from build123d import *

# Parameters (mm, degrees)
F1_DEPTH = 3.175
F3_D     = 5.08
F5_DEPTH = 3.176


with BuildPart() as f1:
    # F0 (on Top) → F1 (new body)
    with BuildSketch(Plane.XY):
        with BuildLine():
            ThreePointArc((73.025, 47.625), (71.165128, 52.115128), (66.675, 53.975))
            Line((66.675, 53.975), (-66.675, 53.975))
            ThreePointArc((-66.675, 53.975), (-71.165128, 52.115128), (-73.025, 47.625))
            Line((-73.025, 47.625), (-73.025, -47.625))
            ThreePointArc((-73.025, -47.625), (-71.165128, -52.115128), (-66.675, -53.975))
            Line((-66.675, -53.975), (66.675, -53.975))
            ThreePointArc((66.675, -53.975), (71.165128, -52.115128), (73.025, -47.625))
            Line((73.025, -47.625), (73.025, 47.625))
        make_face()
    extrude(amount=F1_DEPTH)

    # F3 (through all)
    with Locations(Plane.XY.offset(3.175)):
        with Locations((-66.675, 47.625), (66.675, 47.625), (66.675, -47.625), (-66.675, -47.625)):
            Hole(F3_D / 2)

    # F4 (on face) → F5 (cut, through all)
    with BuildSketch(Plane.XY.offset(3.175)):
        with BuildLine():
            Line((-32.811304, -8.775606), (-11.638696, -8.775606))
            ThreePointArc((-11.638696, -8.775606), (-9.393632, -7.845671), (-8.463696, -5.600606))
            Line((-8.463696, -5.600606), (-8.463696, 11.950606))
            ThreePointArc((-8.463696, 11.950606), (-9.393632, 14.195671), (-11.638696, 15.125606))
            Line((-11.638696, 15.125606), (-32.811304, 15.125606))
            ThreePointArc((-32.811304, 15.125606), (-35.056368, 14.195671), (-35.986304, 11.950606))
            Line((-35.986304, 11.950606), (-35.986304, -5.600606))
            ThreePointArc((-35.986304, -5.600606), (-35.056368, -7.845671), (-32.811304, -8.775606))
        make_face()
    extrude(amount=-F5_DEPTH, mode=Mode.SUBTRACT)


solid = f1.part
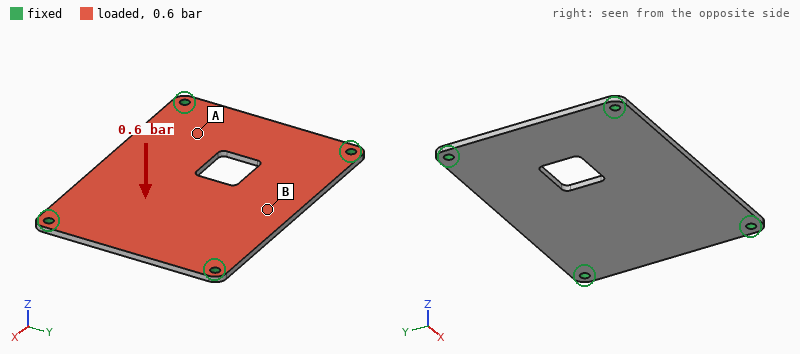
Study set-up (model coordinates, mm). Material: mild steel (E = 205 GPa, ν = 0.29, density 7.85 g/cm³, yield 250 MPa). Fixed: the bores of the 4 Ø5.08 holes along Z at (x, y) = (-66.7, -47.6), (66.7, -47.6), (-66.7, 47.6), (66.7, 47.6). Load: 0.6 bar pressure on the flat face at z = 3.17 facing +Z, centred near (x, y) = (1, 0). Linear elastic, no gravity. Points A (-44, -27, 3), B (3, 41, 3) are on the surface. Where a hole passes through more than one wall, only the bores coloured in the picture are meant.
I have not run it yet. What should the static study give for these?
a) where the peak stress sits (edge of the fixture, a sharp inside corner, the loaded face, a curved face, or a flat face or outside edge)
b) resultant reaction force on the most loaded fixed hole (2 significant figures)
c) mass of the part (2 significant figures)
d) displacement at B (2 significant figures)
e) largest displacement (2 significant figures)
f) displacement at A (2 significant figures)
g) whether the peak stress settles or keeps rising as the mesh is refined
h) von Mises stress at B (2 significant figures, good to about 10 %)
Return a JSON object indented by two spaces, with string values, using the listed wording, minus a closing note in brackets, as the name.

{
  "where the peak stress sits": "edge of the fixture",
  "resultant reaction force on the most loaded fixed hole": "230 N",
  "mass of the part": "370 g",
  "displacement at B": "0.14 mm",
  "largest displacement": "0.17 mm",
  "displacement at A": "0.075 mm",
  "whether the peak stress settles or keeps rising as the mesh is refined": "keeps rising",
  "von Mises stress at B": "33 MPa"
}
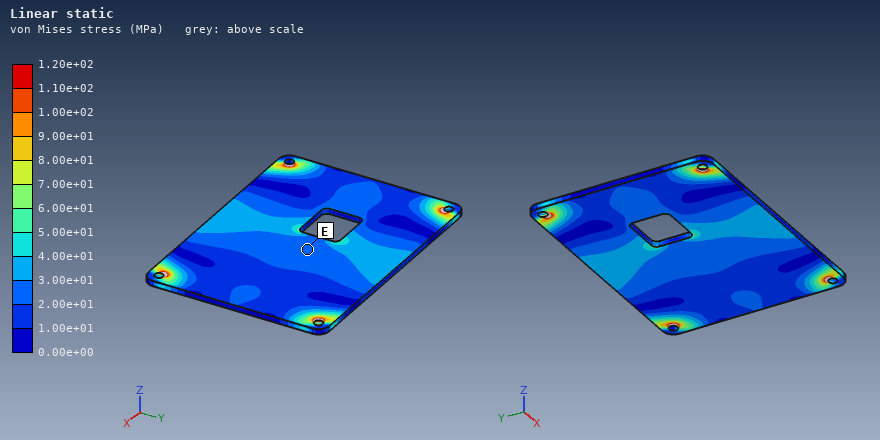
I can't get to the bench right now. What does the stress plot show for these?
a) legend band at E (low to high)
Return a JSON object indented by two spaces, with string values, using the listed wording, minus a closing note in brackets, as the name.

{
  "legend band at E": "2.00e+01 to 3.00e+01 MPa"
}
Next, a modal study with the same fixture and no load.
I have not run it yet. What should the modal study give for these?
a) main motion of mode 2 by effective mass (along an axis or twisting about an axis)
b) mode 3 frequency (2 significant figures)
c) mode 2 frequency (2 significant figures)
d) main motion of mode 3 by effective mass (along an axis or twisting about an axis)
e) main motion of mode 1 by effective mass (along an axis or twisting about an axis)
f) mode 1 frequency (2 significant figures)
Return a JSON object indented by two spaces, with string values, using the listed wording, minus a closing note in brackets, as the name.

{
  "main motion of mode 2 by effective mass": "twisting about X",
  "mode 3 frequency": "1700 Hz",
  "mode 2 frequency": "1200 Hz",
  "main motion of mode 3 by effective mass": "twisting about Y",
  "main motion of mode 1 by effective mass": "along Z",
  "mode 1 frequency": "720 Hz"
}
